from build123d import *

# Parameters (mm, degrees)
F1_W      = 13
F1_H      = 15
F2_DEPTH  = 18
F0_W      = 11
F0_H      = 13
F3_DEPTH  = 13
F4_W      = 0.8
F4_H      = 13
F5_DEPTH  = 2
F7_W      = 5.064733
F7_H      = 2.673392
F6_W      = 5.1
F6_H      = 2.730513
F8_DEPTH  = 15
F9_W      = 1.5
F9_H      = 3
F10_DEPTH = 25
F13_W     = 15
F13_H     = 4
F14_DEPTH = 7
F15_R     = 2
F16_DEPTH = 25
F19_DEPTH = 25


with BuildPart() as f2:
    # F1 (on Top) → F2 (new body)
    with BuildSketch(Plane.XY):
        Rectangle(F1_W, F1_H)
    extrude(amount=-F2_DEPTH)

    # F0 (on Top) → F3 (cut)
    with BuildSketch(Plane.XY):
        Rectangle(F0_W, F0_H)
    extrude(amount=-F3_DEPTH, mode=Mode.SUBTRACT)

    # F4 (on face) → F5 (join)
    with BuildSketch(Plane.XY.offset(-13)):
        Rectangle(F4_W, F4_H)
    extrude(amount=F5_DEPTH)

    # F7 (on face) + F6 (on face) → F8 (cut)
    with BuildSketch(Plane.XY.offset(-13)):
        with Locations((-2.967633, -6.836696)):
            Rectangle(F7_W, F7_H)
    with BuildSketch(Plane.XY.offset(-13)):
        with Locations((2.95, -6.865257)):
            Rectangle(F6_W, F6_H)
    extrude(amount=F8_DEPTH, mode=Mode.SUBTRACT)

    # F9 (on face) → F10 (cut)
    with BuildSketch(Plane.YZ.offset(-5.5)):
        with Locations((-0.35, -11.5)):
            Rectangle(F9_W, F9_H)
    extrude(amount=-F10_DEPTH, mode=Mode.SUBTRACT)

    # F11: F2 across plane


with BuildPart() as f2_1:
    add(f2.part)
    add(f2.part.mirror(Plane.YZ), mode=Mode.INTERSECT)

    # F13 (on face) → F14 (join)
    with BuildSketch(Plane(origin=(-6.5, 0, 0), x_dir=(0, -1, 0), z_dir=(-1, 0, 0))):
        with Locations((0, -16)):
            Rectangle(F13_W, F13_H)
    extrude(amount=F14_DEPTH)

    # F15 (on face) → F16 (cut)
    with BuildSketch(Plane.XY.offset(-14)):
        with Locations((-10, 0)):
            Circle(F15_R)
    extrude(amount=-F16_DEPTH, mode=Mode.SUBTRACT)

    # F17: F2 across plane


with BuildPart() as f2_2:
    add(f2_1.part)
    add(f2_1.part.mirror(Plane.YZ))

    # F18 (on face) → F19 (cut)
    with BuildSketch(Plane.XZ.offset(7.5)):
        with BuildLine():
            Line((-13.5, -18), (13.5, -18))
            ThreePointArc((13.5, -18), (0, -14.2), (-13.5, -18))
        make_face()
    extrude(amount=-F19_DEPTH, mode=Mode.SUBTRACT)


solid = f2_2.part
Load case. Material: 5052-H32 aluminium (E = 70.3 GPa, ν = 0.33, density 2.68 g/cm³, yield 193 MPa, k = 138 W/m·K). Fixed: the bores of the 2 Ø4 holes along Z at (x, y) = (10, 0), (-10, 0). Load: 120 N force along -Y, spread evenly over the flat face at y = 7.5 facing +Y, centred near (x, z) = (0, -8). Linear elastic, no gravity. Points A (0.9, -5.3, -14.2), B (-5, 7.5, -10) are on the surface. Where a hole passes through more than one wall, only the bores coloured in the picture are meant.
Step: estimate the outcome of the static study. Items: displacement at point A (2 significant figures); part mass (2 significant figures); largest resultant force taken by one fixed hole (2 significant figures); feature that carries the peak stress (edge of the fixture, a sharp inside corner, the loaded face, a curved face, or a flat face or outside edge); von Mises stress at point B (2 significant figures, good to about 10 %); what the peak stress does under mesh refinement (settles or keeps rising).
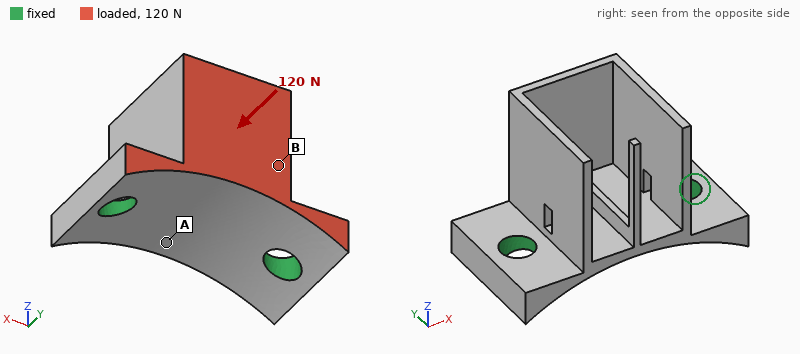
6.1 µm
3.4 g
60 N
edge of the fixture
14 MPa
keeps rising
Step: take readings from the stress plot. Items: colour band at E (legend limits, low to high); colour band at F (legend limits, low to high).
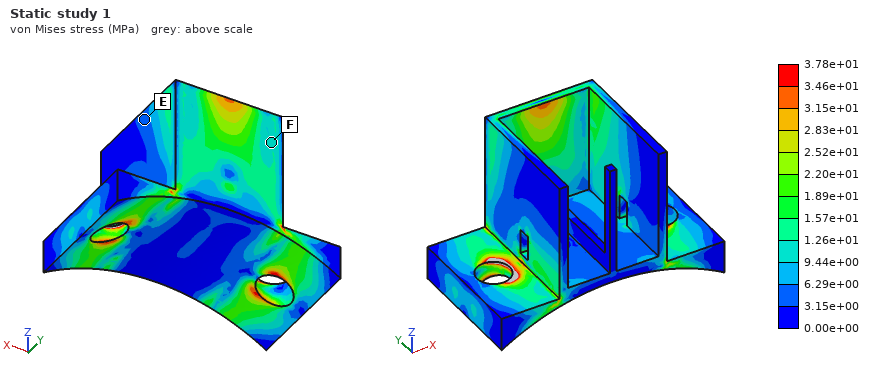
3.15e+00 to 6.29e+00 MPa
9.44e+00 to 1.26e+01 MPa
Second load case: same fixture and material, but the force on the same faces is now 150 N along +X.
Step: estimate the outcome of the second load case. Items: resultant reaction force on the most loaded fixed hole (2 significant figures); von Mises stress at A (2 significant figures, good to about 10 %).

110 N
6.8 MPa
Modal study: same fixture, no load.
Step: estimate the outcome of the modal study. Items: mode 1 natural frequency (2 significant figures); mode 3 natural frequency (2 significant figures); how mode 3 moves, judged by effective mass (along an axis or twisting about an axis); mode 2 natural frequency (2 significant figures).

4400 Hz
7000 Hz
along X
6000 Hz
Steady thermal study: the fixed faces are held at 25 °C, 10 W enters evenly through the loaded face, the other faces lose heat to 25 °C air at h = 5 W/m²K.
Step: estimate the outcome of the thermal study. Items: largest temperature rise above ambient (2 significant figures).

26 K
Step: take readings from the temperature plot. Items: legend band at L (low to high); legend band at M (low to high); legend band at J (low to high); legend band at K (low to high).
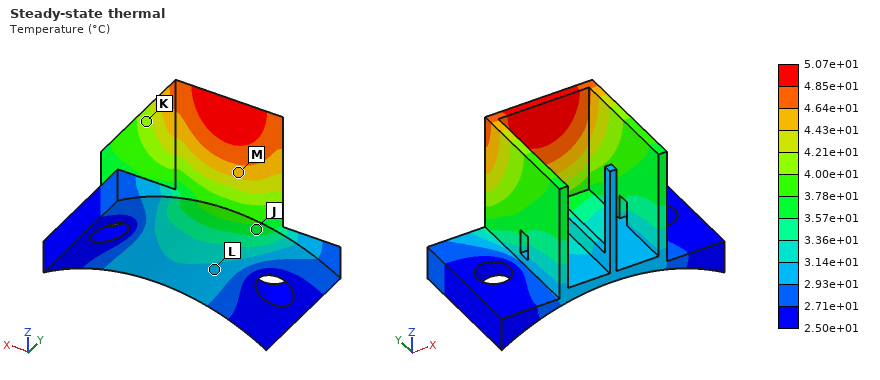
2.93e+01 to 3.14e+01 °C
4.43e+01 to 4.64e+01 °C
3.57e+01 to 3.78e+01 °C
4.00e+01 to 4.21e+01 °C
